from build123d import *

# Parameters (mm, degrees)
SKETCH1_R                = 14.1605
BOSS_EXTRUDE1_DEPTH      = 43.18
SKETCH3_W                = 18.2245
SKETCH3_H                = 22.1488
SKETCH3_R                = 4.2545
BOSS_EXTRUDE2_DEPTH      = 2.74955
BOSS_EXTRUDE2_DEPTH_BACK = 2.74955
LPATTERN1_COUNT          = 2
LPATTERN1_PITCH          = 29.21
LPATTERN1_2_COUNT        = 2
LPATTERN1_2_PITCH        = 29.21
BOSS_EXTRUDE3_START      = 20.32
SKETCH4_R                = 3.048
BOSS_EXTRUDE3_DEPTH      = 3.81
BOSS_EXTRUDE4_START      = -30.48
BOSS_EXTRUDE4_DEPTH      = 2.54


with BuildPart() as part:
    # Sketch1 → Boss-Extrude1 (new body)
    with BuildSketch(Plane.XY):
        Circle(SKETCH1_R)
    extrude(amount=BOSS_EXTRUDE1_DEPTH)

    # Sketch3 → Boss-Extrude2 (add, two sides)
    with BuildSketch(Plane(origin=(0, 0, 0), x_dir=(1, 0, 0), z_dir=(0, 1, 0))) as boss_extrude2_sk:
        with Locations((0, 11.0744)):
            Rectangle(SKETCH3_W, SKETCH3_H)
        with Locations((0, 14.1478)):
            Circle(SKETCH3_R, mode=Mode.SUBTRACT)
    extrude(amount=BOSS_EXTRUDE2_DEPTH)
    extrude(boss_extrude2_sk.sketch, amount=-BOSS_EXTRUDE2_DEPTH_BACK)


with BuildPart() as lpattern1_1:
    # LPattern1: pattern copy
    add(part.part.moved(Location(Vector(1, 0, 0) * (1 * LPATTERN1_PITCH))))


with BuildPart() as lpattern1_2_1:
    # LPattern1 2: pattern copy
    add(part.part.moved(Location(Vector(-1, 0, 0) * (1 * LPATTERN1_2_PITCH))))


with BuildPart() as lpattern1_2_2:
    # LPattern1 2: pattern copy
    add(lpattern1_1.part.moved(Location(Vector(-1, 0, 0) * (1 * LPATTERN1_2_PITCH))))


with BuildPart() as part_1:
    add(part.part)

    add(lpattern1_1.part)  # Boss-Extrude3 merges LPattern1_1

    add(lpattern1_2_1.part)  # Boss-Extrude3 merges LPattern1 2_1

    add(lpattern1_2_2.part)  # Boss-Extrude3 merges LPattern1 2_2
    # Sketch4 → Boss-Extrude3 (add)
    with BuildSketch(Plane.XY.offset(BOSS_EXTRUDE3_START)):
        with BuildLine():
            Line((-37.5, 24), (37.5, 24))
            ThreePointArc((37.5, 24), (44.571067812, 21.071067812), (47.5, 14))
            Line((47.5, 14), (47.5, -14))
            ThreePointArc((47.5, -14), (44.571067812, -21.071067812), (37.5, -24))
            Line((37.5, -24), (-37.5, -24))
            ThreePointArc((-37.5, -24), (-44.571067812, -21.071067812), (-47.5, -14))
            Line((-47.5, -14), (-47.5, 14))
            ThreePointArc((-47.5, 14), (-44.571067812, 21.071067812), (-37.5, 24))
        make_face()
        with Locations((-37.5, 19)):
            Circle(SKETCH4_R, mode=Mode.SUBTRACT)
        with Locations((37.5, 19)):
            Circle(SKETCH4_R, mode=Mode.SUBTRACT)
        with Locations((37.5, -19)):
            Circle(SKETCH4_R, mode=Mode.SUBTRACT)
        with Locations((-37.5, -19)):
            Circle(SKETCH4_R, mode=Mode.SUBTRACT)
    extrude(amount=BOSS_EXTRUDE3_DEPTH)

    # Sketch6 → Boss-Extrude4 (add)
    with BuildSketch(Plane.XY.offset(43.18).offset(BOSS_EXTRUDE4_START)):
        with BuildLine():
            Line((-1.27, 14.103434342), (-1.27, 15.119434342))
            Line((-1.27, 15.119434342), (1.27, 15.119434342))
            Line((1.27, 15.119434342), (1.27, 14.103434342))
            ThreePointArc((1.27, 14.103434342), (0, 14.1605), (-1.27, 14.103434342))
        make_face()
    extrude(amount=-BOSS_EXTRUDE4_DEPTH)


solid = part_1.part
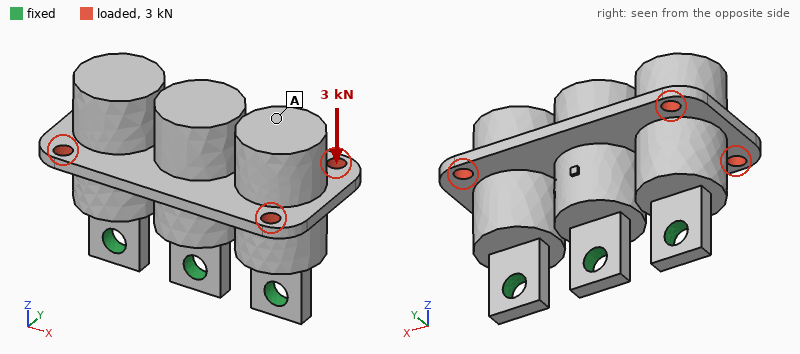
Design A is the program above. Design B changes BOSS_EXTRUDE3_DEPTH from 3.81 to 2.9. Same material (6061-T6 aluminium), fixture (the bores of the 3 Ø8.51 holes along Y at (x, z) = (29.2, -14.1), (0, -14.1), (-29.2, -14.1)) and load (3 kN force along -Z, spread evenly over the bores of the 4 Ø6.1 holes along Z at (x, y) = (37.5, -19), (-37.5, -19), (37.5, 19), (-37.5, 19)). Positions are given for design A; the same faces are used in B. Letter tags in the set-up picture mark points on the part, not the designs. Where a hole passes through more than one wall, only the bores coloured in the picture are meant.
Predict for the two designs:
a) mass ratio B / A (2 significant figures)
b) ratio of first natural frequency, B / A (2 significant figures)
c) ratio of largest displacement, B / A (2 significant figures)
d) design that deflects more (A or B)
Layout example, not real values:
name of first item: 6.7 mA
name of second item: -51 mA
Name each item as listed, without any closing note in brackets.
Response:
mass ratio B / A: 0.98
ratio of first natural frequency, B / A: 1.0
ratio of largest displacement, B / A: 1.9
design that deflects more: B
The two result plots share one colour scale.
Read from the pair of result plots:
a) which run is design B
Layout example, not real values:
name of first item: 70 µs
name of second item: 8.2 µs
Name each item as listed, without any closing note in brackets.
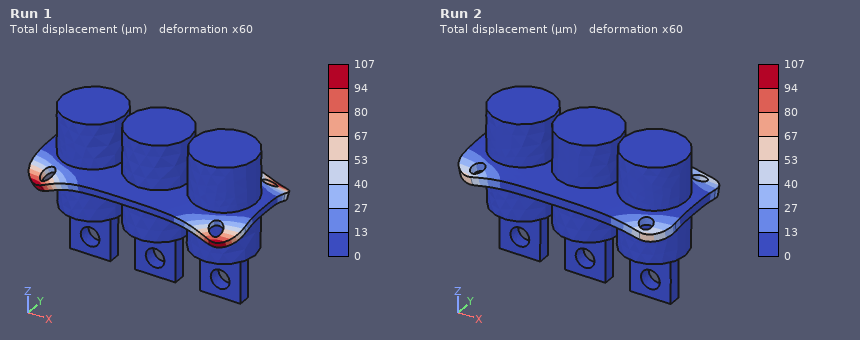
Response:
which run is design B: Run 1
